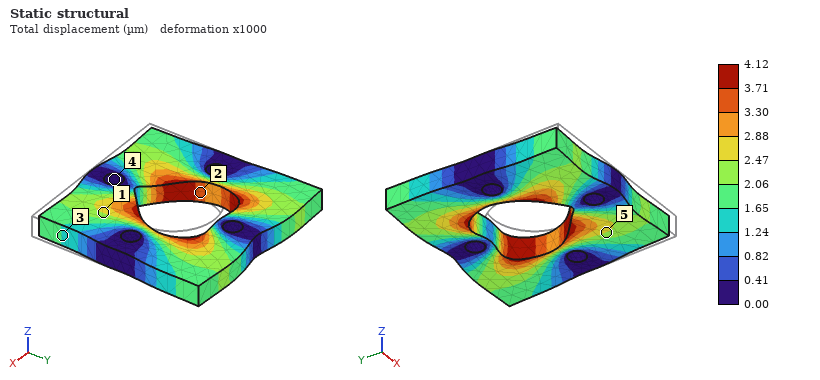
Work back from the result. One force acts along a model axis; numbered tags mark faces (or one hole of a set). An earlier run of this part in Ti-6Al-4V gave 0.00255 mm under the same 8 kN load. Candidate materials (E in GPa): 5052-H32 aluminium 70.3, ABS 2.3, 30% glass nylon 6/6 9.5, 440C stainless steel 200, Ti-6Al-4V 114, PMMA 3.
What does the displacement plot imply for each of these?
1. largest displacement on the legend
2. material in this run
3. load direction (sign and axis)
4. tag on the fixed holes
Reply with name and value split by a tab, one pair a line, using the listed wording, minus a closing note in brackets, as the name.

largest displacement on the legend	4.12 µm
material in this run	5052-H32 aluminium
load direction	+Y
tag on the fixed holes	4
